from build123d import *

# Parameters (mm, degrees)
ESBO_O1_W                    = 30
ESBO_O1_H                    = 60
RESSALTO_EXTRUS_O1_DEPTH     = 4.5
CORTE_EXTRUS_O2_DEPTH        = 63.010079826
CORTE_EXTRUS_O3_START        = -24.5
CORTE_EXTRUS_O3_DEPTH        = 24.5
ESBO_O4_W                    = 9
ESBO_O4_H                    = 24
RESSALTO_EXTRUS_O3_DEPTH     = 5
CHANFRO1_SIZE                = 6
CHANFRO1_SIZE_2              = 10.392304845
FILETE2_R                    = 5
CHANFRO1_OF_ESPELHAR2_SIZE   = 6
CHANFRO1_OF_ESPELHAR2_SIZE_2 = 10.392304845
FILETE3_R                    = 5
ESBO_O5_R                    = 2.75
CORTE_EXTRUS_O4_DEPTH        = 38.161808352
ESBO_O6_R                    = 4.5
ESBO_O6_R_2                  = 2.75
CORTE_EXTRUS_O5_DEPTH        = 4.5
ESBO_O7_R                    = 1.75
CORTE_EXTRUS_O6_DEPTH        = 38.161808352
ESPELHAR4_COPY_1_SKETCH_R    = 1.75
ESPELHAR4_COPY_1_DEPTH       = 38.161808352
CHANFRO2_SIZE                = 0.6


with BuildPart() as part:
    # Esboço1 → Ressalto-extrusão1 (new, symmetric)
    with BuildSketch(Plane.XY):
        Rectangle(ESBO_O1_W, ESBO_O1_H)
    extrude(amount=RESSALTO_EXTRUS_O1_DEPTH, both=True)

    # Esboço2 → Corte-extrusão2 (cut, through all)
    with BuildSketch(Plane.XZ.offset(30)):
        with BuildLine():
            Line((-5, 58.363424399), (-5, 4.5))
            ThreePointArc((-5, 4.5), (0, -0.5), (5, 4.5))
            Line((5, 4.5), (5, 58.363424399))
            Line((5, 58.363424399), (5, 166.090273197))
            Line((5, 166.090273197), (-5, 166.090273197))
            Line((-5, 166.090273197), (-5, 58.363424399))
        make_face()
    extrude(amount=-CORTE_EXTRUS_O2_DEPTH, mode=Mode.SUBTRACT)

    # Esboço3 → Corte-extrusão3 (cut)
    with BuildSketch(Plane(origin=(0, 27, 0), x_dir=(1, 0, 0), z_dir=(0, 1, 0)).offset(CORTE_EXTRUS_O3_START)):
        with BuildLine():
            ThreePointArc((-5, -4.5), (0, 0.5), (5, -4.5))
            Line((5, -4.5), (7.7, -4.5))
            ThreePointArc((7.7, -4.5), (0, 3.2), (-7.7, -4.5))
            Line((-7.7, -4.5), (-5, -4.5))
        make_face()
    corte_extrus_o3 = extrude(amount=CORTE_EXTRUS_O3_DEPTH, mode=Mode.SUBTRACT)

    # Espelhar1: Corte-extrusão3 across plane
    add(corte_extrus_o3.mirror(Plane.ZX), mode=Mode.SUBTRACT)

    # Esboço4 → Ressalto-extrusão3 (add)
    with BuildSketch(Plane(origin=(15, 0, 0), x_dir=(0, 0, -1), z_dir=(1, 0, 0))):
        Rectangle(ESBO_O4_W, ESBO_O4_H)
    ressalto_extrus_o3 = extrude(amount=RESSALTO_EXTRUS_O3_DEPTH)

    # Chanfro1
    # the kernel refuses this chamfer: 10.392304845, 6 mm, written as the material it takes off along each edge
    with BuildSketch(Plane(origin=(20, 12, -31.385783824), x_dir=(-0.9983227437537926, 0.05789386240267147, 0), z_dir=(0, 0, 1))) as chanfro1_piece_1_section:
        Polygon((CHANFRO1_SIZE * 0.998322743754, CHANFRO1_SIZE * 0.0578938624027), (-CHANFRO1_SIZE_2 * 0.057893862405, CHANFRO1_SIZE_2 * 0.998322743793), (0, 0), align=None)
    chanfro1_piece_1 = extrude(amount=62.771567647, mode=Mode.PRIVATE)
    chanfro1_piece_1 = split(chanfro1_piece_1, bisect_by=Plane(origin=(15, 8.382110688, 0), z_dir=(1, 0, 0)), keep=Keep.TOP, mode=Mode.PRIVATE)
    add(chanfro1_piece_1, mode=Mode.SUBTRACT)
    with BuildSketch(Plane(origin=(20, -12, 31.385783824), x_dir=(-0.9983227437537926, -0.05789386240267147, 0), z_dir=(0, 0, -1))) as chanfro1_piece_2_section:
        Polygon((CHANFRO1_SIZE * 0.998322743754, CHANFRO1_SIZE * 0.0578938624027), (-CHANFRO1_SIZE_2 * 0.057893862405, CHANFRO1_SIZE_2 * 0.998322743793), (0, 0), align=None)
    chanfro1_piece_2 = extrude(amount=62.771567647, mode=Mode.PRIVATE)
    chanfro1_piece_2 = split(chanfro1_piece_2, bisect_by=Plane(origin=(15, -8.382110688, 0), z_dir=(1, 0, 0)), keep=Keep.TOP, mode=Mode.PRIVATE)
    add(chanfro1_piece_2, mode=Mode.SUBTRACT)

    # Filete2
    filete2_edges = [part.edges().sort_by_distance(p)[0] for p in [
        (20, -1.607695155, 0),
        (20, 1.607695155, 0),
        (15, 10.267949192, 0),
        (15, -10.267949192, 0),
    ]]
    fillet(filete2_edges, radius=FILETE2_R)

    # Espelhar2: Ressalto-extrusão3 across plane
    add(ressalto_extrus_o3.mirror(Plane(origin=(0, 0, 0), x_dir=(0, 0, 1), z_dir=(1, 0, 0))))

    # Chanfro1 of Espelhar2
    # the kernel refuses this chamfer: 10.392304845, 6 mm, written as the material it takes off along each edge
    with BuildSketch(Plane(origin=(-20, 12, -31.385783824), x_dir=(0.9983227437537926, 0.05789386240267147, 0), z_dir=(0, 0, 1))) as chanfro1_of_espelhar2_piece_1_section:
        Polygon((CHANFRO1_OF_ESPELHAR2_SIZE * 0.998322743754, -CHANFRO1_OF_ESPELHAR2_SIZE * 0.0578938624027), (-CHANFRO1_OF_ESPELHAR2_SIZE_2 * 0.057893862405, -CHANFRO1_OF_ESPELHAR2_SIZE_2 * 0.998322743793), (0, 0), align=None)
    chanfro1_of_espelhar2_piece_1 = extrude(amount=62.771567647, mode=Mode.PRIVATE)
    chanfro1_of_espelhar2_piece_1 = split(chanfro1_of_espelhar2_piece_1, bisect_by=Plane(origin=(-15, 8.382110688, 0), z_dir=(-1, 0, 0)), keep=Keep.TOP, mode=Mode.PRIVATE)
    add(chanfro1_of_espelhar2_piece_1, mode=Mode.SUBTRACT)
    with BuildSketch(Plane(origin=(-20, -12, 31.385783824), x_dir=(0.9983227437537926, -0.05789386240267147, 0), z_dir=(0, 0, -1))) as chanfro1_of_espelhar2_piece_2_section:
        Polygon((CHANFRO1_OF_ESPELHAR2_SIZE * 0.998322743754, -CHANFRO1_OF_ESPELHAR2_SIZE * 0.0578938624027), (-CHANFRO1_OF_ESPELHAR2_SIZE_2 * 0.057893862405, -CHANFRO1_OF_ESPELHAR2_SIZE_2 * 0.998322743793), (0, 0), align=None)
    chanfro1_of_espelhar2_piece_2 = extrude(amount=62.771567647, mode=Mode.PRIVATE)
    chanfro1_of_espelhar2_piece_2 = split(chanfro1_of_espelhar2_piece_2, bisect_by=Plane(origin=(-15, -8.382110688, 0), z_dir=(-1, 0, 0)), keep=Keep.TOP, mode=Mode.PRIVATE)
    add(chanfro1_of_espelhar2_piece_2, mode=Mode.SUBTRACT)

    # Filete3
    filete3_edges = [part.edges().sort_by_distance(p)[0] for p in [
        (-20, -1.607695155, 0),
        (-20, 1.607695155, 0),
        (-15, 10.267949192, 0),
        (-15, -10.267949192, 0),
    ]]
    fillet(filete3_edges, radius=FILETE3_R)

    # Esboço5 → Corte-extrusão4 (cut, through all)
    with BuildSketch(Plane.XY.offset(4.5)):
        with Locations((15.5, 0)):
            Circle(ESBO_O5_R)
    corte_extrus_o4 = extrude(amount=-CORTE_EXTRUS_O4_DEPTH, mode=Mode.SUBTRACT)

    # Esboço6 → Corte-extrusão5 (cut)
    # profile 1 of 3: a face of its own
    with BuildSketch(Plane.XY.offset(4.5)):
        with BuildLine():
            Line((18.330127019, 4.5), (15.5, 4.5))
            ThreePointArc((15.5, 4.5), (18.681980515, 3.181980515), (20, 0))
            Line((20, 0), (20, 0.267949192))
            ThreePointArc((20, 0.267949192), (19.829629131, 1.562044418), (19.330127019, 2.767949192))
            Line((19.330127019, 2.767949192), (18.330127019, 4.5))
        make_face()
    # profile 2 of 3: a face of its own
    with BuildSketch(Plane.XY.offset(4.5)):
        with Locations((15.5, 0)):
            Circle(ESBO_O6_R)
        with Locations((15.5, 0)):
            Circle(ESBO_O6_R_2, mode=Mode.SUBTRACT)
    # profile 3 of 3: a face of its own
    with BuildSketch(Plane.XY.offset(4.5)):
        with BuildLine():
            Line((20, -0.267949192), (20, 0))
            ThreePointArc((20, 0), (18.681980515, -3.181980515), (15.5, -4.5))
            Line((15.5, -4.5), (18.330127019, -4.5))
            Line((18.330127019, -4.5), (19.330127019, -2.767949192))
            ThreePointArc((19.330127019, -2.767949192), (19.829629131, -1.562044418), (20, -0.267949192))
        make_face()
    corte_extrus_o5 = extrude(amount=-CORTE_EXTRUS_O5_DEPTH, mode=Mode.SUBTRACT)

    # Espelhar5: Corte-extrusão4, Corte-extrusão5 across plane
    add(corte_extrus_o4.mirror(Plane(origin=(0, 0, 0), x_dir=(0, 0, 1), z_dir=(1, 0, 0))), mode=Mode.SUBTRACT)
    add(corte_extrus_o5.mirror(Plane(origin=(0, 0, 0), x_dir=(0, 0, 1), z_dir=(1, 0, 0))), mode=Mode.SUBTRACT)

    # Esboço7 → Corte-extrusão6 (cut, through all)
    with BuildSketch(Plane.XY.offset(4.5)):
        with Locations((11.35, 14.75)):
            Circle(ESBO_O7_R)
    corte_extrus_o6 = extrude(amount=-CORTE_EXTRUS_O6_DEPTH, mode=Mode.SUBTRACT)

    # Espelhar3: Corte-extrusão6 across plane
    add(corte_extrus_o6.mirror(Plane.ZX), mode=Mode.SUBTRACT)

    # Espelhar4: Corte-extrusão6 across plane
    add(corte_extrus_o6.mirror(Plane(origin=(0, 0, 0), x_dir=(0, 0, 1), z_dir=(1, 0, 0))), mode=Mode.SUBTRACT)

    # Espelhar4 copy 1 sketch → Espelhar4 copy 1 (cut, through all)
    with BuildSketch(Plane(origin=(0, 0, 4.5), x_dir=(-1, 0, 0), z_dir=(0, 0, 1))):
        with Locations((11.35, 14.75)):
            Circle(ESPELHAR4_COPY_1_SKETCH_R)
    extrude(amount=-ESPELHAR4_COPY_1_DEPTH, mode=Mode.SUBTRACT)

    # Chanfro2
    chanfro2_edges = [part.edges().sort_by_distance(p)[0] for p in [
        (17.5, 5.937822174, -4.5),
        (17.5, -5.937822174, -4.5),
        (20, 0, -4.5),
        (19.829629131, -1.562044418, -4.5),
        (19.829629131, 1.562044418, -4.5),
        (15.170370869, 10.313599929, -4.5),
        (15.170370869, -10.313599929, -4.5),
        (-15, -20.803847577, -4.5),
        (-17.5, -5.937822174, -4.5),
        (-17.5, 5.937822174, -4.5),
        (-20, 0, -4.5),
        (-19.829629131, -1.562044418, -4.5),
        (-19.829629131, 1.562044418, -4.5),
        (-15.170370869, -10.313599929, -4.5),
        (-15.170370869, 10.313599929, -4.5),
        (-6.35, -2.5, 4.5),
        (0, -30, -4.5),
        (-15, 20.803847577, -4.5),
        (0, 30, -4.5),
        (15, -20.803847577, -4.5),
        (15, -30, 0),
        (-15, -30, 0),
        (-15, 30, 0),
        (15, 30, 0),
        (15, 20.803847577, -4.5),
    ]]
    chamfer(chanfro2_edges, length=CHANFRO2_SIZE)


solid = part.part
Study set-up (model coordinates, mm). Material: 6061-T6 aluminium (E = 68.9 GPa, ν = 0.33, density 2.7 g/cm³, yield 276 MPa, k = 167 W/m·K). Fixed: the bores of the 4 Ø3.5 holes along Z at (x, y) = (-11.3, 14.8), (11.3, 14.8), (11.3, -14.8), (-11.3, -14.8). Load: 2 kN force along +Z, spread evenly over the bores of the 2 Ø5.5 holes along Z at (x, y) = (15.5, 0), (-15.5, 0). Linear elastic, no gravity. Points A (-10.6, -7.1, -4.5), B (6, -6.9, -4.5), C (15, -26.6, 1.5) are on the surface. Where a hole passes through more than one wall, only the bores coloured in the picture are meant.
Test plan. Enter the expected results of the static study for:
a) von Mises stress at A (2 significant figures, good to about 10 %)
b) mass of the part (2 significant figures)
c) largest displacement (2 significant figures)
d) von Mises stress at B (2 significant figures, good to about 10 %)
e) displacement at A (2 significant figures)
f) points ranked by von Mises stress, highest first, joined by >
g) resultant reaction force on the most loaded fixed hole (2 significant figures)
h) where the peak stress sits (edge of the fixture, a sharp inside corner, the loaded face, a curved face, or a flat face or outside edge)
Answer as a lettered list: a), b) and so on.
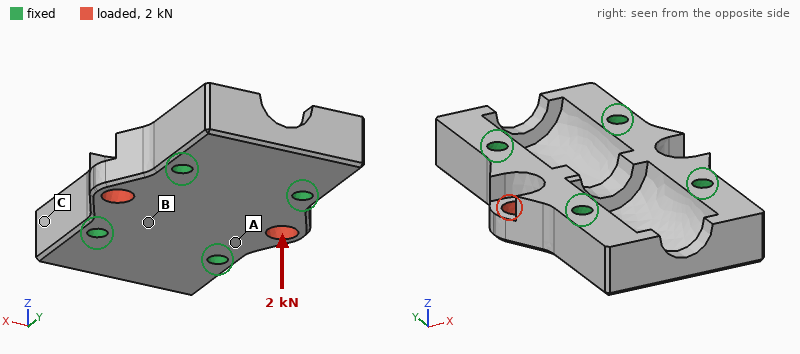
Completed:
a) 20 MPa
b) 30 g
c) 20 µm
d) 12 MPa
e) 4.1 µm
f) A > B > C
g) 520 N
h) the loaded face
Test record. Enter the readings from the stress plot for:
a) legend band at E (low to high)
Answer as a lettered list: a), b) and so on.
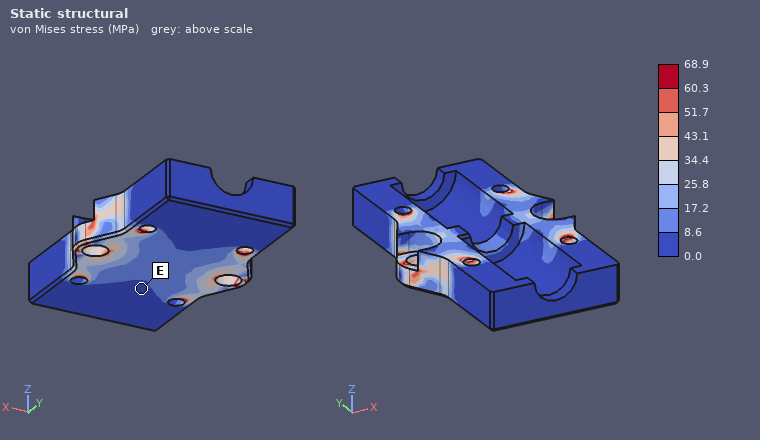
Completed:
a) 0.0 to 8.6 MPa
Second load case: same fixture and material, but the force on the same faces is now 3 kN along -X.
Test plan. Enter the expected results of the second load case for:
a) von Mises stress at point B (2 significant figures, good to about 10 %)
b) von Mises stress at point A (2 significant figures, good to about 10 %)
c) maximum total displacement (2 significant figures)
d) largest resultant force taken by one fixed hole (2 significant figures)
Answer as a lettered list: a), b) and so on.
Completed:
a) 22 MPa
b) 25 MPa
c) 12 µm
d) 770 N
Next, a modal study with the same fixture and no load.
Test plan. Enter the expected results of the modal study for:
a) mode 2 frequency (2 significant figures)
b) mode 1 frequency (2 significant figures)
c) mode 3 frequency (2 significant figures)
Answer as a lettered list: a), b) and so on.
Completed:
a) 24 kHz
b) 23 kHz
c) 27 kHz
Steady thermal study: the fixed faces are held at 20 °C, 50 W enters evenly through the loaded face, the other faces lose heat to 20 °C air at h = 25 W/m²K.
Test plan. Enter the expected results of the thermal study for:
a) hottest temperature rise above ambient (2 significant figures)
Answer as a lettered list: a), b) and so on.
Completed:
a) 23 K
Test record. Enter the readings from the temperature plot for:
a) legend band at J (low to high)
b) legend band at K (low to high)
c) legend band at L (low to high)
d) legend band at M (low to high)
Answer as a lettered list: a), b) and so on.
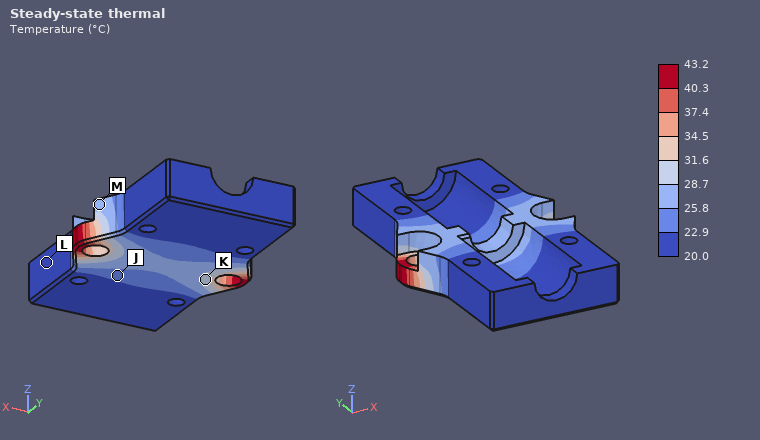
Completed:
a) 22.9 to 25.8 °C
b) 28.7 to 31.6 °C
c) 20.0 to 22.9 °C
d) 25.8 to 28.7 °C
